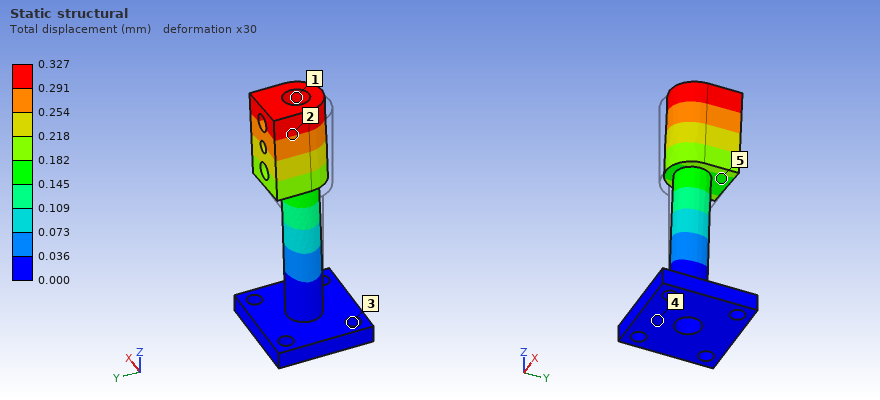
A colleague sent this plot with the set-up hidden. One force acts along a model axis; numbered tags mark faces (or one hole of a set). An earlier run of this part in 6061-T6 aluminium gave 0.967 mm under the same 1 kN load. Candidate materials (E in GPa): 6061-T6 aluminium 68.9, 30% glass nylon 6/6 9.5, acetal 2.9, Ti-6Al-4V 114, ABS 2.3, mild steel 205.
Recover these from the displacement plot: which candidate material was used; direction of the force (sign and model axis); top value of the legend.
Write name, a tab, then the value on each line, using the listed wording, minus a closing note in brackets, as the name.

which candidate material was used	mild steel
direction of the force	+X
top value of the legend	0.327 mm
